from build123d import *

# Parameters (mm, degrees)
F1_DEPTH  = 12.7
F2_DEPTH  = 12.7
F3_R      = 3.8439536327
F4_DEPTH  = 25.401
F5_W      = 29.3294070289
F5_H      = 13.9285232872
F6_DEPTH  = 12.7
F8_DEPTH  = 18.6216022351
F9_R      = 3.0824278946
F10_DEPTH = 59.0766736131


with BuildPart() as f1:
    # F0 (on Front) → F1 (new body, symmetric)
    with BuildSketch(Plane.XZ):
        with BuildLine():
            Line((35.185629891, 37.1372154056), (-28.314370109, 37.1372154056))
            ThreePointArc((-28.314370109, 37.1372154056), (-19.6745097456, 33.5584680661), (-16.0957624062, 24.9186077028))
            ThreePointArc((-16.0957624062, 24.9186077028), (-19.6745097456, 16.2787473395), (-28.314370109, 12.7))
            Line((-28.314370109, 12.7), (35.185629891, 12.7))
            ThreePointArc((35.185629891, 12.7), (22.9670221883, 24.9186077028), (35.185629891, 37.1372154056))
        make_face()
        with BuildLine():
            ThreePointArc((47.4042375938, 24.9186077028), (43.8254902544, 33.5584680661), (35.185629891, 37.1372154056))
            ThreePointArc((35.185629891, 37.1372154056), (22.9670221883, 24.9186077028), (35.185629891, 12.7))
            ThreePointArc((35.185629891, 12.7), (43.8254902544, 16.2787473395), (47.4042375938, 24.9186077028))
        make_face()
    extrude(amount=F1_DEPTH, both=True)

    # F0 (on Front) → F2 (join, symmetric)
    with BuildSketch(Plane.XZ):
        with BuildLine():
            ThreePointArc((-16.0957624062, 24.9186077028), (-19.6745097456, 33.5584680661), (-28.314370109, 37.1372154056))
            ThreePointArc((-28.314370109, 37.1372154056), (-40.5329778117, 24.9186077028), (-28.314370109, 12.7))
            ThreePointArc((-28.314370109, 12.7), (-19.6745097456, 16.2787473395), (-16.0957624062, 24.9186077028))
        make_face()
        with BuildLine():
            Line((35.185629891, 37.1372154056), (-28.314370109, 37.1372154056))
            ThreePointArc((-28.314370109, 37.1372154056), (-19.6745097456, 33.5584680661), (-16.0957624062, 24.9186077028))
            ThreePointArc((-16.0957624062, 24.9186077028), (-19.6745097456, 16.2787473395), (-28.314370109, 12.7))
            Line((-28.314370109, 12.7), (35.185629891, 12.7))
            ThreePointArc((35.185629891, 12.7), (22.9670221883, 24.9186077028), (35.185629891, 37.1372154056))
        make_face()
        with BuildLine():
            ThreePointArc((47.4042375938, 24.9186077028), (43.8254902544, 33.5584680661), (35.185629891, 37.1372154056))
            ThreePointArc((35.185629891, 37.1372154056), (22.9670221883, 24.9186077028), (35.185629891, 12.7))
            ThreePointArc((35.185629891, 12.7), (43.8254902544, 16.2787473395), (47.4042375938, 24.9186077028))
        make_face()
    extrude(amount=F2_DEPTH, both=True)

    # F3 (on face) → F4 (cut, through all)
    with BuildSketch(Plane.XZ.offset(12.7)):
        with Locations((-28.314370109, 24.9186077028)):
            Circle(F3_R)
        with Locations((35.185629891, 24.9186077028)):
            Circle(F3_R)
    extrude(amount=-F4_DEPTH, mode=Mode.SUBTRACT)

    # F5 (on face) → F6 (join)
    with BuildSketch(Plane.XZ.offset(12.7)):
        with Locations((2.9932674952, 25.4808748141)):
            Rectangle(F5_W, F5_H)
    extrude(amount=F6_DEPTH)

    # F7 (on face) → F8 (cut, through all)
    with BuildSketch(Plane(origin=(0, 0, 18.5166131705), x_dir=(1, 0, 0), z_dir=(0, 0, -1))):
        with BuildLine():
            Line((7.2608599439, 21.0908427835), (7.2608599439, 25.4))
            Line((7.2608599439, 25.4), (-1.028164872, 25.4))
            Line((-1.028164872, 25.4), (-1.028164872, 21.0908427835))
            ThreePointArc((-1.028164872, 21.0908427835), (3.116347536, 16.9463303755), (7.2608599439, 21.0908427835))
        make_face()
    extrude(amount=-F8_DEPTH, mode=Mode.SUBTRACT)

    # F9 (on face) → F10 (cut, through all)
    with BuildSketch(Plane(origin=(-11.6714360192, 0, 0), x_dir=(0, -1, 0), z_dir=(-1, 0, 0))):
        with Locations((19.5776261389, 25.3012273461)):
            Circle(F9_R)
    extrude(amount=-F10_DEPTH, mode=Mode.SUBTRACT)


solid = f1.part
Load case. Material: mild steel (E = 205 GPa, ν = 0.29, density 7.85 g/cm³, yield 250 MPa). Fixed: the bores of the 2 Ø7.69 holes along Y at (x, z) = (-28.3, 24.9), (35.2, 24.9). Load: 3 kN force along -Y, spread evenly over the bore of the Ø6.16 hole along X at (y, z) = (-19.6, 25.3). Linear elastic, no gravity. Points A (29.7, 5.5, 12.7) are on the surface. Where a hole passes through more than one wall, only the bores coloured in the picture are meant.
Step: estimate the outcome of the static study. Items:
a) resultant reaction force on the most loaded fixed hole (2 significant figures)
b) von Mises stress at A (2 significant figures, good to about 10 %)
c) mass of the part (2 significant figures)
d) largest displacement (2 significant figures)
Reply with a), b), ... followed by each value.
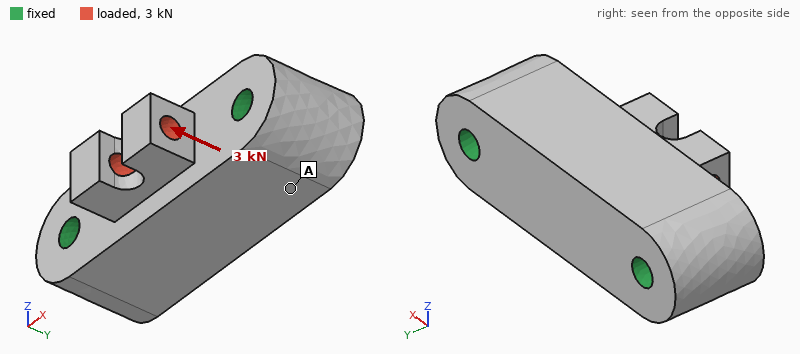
a) 1.5 kN
b) 2.7 MPa
c) 410 g
d) 2.1 µm
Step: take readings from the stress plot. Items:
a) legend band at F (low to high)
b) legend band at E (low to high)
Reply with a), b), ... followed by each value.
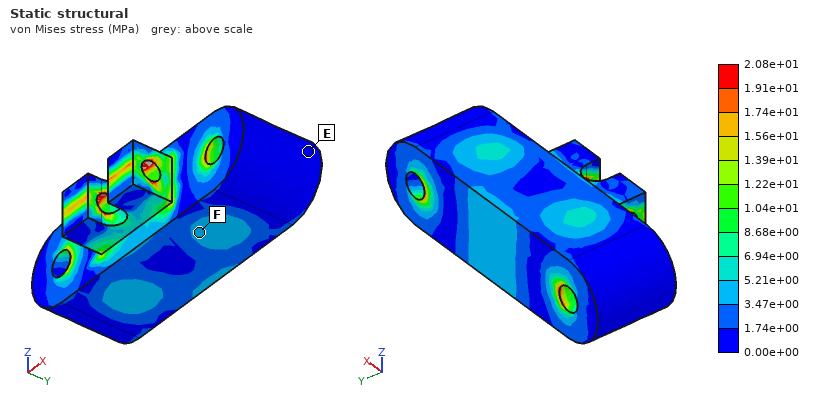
a) 3.47e+00 to 5.21e+00 MPa
b) 0.00e+00 to 1.74e+00 MPa
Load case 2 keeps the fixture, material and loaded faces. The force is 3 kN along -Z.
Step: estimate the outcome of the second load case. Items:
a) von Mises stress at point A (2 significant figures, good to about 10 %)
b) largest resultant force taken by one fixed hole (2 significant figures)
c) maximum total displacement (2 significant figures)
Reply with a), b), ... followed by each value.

a) 10 MPa
b) 1.5 kN
c) 9.4 µm
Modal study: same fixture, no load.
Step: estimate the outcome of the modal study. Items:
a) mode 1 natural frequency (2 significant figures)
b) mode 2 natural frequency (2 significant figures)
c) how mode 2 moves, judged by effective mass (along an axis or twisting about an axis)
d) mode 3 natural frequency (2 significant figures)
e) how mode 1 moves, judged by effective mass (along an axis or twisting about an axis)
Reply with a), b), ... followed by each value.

a) 14 kHz
b) 18 kHz
c) along Y
d) 19 kHz
e) along Z
